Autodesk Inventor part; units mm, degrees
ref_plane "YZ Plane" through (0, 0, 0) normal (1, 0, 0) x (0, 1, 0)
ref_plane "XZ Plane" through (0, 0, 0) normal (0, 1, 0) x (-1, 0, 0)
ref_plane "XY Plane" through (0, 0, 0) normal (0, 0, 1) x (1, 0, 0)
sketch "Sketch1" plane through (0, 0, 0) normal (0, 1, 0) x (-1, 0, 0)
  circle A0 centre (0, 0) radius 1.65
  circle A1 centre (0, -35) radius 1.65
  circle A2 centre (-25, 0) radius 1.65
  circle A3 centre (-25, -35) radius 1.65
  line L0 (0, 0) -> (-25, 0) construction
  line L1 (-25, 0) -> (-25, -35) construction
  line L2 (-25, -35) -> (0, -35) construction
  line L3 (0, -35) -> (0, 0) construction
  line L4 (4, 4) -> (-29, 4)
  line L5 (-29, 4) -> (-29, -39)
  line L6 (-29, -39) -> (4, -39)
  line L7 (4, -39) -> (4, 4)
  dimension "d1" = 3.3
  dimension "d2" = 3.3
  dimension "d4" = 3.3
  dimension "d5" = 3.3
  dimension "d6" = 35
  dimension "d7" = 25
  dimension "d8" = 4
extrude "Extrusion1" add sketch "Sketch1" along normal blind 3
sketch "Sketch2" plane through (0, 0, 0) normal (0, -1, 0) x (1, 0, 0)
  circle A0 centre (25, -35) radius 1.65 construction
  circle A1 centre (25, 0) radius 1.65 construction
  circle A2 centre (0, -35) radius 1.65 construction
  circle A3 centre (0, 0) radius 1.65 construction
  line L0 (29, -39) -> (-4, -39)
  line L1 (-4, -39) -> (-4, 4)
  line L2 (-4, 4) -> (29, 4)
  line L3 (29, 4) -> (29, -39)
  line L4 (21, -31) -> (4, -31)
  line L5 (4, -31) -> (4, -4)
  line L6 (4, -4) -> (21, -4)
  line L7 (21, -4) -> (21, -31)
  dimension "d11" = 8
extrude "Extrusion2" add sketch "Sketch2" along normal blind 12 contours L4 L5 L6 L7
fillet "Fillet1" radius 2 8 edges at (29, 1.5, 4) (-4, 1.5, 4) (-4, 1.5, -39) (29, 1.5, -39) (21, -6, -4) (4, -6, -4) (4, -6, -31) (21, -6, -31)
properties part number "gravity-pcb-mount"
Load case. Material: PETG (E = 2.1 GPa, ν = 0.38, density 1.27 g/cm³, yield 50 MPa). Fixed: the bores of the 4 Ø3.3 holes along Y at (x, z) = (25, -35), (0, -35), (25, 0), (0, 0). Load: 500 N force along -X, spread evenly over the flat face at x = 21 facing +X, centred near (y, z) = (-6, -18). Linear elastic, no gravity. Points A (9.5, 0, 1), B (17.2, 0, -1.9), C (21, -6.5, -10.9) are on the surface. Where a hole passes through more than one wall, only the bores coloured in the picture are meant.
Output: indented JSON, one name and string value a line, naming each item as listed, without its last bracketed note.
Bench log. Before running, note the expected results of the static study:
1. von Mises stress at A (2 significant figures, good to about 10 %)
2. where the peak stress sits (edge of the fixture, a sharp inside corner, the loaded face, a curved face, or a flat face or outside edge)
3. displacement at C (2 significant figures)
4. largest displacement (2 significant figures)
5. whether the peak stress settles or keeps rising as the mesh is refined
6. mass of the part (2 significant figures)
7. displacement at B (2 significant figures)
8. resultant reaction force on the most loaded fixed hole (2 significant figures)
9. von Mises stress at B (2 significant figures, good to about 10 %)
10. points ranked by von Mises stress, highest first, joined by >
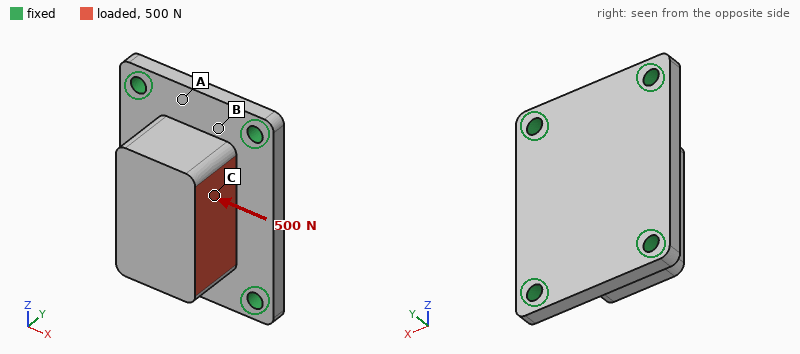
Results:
{
  "von Mises stress at A": "5.2 MPa",
  "where the peak stress sits": "edge of the fixture",
  "displacement at C": "0.16 mm",
  "largest displacement": "0.22 mm",
  "whether the peak stress settles or keeps rising as the mesh is refined": "keeps rising",
  "mass of the part": "12 g",
  "displacement at B": "0.034 mm",
  "resultant reaction force on the most loaded fixed hole": "170 N",
  "von Mises stress at B": "9.2 MPa",
  "points ranked by von Mises stress, highest first, joined by >": "B > A > C"
}
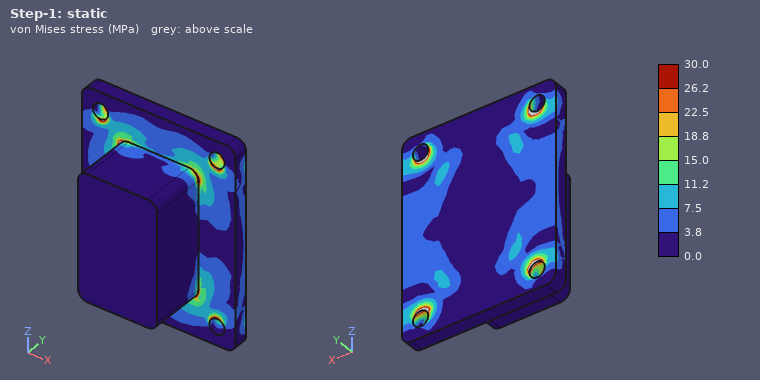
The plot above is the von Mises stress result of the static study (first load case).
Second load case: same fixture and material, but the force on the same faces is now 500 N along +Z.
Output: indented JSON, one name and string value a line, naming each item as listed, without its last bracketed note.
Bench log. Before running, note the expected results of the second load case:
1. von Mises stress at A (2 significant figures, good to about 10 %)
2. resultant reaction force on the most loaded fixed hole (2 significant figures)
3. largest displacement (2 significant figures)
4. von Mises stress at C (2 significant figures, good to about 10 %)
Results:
{
  "von Mises stress at A": "4.3 MPa",
  "resultant reaction force on the most loaded fixed hole": "170 N",
  "largest displacement": "0.14 mm",
  "von Mises stress at C": "4.4 MPa"
}
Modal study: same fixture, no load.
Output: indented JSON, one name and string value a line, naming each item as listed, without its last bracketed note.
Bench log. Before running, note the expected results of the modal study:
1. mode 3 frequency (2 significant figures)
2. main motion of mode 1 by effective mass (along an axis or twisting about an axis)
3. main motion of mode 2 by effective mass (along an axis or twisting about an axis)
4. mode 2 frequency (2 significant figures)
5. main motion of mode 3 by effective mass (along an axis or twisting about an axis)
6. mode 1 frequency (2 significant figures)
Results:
{
  "mode 3 frequency": "3900 Hz",
  "main motion of mode 1 by effective mass": "along Y",
  "main motion of mode 2 by effective mass": "along X",
  "mode 2 frequency": "3000 Hz",
  "main motion of mode 3 by effective mass": "along Z",
  "mode 1 frequency": "2800 Hz"
}
